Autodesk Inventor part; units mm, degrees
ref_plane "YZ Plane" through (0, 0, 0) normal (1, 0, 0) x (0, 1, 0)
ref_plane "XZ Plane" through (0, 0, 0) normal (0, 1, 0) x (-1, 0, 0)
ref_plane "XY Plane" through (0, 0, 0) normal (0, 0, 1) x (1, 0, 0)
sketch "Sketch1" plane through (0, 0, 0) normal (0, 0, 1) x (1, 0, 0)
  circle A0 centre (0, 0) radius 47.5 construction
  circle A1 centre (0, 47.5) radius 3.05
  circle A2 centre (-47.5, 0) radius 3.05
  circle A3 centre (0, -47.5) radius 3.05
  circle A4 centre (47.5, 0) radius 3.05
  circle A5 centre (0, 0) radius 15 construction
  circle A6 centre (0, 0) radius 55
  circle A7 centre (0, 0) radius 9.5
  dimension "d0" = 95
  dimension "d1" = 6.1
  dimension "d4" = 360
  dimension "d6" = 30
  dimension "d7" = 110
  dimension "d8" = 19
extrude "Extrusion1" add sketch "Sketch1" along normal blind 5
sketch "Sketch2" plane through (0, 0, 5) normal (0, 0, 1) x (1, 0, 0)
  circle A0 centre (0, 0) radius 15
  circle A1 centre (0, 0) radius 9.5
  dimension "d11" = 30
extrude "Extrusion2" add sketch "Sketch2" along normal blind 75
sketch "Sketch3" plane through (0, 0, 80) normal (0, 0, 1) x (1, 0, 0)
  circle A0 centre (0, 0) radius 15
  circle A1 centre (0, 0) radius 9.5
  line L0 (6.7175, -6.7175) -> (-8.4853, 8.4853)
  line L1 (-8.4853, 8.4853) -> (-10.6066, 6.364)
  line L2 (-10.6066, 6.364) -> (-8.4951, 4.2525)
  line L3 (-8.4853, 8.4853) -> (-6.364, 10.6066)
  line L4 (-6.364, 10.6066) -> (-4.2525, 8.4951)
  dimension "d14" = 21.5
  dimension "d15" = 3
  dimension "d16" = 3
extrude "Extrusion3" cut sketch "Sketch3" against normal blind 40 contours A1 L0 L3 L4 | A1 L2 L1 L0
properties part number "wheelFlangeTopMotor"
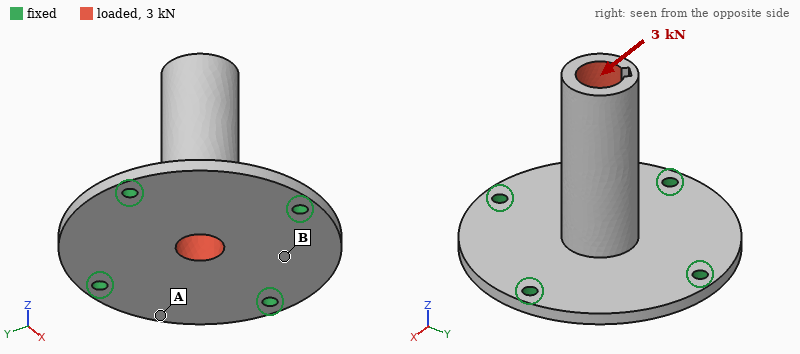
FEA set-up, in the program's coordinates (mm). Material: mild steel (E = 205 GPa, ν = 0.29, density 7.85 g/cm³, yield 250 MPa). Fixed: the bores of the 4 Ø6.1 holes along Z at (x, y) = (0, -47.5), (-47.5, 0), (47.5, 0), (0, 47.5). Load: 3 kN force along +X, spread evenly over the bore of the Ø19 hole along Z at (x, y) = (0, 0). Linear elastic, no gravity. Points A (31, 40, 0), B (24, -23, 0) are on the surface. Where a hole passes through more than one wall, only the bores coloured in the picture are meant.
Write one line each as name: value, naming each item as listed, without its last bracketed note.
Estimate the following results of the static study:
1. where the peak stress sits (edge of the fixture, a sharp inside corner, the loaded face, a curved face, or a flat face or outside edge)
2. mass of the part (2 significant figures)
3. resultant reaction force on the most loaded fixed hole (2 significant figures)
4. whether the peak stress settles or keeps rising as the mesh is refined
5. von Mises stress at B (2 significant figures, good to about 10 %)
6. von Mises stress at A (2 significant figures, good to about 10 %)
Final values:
where the peak stress sits: edge of the fixture
mass of the part: 600 g
resultant reaction force on the most loaded fixed hole: 1.7 kN
whether the peak stress settles or keeps rising as the mesh is refined: keeps rising
von Mises stress at B: 44 MPa
von Mises stress at A: 22 MPa
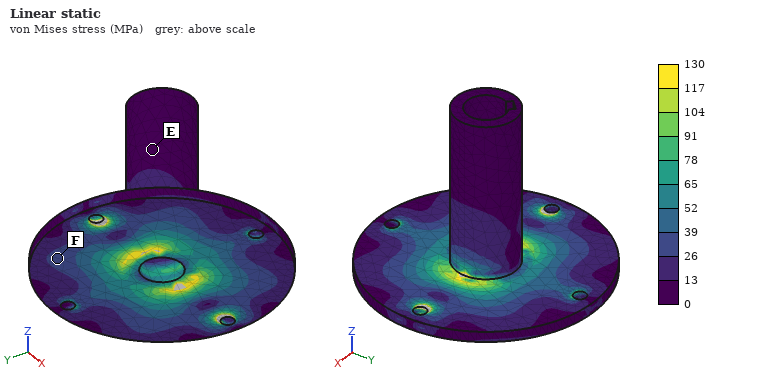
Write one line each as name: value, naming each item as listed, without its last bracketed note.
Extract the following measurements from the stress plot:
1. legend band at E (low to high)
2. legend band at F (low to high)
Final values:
legend band at E: 0 to 13 MPa
legend band at F: 26 to 39 MPa
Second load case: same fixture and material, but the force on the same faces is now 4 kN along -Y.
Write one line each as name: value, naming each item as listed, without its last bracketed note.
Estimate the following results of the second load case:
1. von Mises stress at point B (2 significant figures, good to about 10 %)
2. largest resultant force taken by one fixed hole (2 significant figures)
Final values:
von Mises stress at point B: 58 MPa
largest resultant force taken by one fixed hole: 2.3 kN
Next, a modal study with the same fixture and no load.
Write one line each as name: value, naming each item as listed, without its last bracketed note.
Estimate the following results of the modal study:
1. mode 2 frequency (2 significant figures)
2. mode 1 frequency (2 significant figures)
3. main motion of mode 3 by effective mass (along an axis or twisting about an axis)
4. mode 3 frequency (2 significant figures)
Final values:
mode 2 frequency: 1400 Hz
mode 1 frequency: 1400 Hz
main motion of mode 3 by effective mass: along Z
mode 3 frequency: 2400 Hz
